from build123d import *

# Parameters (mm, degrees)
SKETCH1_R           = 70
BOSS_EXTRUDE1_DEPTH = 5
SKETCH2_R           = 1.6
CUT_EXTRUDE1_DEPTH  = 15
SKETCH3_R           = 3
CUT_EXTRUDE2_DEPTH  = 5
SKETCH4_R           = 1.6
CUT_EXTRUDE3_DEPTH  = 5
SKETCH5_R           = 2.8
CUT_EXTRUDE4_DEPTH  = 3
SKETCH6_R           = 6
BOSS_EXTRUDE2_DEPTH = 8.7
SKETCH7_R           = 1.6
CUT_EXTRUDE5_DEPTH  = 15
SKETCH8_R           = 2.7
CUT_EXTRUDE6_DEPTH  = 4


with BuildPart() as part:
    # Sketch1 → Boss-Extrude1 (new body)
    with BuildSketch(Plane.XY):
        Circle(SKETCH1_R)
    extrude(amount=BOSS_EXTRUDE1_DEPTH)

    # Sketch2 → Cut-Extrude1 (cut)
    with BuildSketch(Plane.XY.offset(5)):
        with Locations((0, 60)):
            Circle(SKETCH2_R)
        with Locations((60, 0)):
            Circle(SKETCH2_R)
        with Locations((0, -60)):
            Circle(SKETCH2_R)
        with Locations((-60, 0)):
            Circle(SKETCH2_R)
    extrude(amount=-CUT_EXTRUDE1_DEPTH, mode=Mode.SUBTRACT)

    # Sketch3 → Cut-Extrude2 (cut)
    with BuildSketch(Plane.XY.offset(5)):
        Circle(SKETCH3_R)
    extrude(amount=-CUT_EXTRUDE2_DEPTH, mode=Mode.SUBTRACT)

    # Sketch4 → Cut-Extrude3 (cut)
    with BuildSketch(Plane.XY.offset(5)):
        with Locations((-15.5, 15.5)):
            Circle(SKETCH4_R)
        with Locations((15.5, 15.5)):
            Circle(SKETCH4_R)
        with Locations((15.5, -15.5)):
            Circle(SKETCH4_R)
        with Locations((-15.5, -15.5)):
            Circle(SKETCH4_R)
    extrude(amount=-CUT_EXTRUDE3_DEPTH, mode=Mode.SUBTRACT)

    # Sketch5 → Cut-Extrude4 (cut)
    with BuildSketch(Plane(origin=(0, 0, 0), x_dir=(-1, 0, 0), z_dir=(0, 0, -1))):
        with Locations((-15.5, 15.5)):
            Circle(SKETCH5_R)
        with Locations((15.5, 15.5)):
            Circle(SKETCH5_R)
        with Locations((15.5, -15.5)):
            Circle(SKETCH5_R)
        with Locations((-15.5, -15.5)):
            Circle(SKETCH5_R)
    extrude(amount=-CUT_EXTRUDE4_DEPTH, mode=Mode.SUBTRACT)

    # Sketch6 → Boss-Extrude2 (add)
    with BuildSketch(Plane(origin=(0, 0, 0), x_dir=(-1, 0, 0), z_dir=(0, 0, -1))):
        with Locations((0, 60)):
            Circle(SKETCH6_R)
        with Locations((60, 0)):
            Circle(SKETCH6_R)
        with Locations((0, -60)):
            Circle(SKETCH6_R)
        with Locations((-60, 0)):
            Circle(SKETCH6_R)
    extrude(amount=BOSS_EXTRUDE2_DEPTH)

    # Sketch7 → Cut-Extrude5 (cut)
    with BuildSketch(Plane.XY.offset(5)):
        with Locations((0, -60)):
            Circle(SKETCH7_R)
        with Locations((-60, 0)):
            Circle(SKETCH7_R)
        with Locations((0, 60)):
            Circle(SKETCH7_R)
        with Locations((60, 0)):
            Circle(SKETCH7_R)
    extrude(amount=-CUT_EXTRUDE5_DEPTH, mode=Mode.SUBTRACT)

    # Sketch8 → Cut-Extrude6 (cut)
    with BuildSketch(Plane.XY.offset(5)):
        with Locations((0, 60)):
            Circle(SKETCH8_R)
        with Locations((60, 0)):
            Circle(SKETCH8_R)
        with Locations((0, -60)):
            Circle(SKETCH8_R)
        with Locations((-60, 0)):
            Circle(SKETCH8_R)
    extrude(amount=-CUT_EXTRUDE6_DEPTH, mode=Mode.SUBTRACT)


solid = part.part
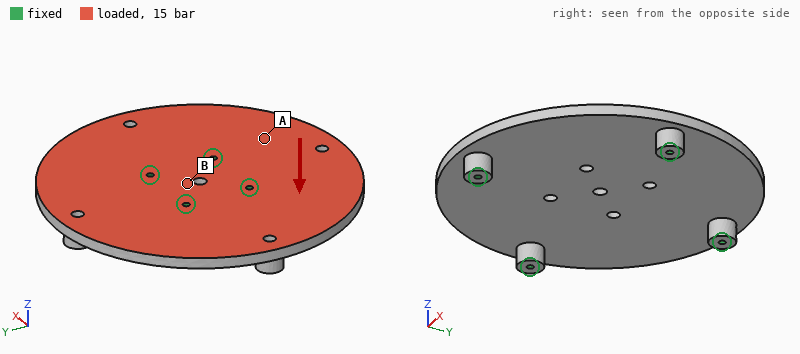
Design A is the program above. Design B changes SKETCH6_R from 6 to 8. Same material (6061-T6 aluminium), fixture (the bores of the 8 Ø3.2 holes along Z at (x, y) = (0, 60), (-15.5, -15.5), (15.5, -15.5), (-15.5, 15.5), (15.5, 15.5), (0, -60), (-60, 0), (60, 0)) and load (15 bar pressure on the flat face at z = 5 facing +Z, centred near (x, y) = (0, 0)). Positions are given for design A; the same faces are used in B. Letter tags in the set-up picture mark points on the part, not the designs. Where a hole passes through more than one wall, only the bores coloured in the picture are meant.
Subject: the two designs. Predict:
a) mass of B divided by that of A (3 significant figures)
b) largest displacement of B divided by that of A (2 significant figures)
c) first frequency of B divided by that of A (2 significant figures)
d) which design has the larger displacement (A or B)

1.04
0.87
1.1
A
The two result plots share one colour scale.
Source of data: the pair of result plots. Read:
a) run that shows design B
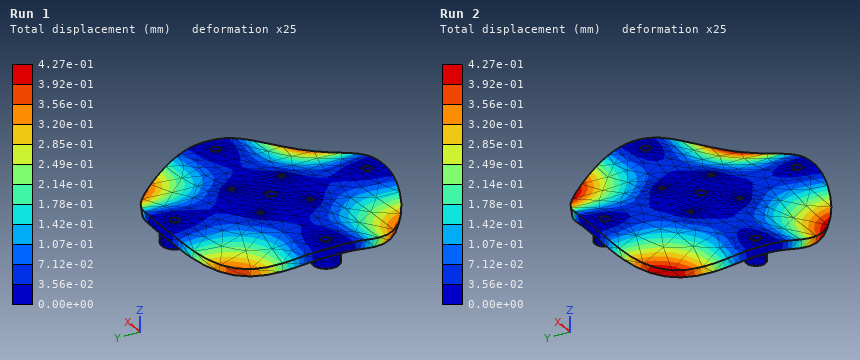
Run 1
